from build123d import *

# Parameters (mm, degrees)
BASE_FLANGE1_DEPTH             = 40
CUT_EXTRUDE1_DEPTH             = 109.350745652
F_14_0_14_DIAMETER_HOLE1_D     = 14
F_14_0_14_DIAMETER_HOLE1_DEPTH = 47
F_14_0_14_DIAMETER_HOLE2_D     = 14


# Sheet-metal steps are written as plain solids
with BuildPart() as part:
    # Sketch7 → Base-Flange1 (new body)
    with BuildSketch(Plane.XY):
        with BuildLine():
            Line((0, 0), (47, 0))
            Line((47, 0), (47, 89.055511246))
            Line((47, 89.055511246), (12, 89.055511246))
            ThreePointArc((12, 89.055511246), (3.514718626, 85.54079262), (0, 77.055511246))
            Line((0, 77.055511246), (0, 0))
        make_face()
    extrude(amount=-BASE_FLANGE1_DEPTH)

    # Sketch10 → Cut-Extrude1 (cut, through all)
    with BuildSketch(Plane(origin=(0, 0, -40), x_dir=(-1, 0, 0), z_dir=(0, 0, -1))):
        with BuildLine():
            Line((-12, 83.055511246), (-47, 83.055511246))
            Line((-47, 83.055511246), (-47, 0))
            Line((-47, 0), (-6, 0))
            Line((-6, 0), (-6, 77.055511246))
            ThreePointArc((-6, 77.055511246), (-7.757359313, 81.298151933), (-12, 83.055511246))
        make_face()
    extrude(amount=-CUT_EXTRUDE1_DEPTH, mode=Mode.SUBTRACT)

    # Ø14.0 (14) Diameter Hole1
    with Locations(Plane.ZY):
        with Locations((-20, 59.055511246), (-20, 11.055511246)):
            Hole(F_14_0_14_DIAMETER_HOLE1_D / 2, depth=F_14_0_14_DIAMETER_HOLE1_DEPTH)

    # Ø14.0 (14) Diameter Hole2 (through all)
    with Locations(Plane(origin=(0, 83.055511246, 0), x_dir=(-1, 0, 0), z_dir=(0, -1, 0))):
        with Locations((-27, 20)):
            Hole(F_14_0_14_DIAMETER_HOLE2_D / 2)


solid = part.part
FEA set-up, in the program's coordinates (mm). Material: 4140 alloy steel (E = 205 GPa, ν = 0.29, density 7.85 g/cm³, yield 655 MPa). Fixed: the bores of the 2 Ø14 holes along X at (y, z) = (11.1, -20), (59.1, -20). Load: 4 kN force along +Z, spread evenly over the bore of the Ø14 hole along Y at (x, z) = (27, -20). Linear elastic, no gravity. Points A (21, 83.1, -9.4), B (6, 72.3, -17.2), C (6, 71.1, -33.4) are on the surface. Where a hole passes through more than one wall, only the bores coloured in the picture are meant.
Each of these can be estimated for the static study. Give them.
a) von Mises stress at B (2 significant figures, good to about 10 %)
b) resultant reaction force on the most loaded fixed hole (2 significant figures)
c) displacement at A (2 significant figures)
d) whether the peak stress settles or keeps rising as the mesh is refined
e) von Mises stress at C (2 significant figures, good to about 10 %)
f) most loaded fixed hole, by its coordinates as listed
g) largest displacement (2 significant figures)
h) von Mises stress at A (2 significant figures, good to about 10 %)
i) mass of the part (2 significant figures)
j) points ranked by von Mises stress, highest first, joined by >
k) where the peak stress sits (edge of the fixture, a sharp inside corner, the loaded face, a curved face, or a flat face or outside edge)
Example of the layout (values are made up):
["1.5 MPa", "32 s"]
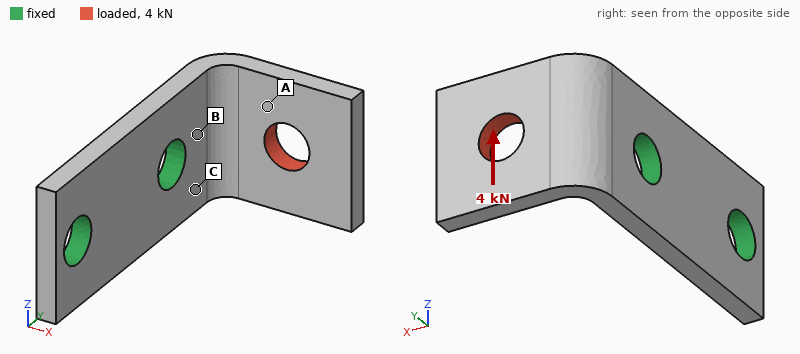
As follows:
["310 MPa", "4.8 kN", "0.15 mm", "keeps rising", "210 MPa", "(59.1, -20)", "0.35 mm", "76 MPa", "220 g", "B > C > A", "edge of the fixture"]
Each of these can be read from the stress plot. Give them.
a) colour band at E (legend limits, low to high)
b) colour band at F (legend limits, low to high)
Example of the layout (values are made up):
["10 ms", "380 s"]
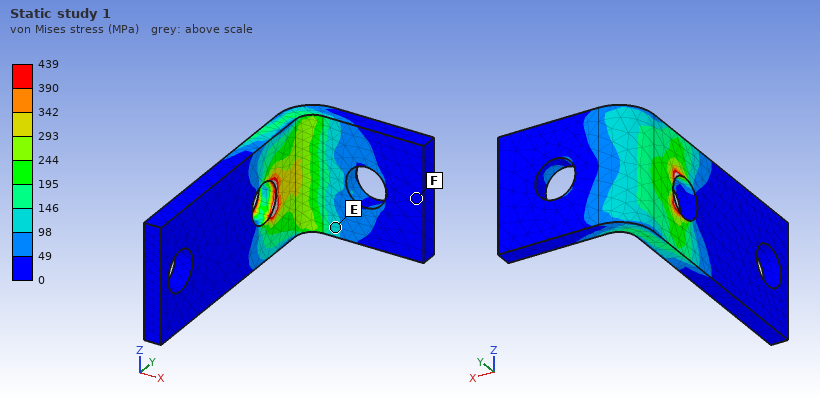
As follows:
["98 to 146 MPa", "0 to 49 MPa"]
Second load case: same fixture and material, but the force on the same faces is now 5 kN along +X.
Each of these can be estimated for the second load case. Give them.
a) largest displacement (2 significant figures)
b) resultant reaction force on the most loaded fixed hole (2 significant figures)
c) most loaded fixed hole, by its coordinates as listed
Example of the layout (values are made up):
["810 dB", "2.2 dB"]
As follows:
["0.42 mm", "5.1 kN", "(59.1, -20)"]
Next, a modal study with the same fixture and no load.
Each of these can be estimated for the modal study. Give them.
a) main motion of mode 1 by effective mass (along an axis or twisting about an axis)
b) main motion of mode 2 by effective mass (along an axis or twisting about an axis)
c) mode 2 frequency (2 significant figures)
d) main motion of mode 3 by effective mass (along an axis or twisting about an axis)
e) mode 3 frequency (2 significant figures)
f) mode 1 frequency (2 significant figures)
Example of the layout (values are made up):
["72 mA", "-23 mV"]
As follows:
["along Y", "along Z", "2300 Hz", "along X", "5000 Hz", "1500 Hz"]
